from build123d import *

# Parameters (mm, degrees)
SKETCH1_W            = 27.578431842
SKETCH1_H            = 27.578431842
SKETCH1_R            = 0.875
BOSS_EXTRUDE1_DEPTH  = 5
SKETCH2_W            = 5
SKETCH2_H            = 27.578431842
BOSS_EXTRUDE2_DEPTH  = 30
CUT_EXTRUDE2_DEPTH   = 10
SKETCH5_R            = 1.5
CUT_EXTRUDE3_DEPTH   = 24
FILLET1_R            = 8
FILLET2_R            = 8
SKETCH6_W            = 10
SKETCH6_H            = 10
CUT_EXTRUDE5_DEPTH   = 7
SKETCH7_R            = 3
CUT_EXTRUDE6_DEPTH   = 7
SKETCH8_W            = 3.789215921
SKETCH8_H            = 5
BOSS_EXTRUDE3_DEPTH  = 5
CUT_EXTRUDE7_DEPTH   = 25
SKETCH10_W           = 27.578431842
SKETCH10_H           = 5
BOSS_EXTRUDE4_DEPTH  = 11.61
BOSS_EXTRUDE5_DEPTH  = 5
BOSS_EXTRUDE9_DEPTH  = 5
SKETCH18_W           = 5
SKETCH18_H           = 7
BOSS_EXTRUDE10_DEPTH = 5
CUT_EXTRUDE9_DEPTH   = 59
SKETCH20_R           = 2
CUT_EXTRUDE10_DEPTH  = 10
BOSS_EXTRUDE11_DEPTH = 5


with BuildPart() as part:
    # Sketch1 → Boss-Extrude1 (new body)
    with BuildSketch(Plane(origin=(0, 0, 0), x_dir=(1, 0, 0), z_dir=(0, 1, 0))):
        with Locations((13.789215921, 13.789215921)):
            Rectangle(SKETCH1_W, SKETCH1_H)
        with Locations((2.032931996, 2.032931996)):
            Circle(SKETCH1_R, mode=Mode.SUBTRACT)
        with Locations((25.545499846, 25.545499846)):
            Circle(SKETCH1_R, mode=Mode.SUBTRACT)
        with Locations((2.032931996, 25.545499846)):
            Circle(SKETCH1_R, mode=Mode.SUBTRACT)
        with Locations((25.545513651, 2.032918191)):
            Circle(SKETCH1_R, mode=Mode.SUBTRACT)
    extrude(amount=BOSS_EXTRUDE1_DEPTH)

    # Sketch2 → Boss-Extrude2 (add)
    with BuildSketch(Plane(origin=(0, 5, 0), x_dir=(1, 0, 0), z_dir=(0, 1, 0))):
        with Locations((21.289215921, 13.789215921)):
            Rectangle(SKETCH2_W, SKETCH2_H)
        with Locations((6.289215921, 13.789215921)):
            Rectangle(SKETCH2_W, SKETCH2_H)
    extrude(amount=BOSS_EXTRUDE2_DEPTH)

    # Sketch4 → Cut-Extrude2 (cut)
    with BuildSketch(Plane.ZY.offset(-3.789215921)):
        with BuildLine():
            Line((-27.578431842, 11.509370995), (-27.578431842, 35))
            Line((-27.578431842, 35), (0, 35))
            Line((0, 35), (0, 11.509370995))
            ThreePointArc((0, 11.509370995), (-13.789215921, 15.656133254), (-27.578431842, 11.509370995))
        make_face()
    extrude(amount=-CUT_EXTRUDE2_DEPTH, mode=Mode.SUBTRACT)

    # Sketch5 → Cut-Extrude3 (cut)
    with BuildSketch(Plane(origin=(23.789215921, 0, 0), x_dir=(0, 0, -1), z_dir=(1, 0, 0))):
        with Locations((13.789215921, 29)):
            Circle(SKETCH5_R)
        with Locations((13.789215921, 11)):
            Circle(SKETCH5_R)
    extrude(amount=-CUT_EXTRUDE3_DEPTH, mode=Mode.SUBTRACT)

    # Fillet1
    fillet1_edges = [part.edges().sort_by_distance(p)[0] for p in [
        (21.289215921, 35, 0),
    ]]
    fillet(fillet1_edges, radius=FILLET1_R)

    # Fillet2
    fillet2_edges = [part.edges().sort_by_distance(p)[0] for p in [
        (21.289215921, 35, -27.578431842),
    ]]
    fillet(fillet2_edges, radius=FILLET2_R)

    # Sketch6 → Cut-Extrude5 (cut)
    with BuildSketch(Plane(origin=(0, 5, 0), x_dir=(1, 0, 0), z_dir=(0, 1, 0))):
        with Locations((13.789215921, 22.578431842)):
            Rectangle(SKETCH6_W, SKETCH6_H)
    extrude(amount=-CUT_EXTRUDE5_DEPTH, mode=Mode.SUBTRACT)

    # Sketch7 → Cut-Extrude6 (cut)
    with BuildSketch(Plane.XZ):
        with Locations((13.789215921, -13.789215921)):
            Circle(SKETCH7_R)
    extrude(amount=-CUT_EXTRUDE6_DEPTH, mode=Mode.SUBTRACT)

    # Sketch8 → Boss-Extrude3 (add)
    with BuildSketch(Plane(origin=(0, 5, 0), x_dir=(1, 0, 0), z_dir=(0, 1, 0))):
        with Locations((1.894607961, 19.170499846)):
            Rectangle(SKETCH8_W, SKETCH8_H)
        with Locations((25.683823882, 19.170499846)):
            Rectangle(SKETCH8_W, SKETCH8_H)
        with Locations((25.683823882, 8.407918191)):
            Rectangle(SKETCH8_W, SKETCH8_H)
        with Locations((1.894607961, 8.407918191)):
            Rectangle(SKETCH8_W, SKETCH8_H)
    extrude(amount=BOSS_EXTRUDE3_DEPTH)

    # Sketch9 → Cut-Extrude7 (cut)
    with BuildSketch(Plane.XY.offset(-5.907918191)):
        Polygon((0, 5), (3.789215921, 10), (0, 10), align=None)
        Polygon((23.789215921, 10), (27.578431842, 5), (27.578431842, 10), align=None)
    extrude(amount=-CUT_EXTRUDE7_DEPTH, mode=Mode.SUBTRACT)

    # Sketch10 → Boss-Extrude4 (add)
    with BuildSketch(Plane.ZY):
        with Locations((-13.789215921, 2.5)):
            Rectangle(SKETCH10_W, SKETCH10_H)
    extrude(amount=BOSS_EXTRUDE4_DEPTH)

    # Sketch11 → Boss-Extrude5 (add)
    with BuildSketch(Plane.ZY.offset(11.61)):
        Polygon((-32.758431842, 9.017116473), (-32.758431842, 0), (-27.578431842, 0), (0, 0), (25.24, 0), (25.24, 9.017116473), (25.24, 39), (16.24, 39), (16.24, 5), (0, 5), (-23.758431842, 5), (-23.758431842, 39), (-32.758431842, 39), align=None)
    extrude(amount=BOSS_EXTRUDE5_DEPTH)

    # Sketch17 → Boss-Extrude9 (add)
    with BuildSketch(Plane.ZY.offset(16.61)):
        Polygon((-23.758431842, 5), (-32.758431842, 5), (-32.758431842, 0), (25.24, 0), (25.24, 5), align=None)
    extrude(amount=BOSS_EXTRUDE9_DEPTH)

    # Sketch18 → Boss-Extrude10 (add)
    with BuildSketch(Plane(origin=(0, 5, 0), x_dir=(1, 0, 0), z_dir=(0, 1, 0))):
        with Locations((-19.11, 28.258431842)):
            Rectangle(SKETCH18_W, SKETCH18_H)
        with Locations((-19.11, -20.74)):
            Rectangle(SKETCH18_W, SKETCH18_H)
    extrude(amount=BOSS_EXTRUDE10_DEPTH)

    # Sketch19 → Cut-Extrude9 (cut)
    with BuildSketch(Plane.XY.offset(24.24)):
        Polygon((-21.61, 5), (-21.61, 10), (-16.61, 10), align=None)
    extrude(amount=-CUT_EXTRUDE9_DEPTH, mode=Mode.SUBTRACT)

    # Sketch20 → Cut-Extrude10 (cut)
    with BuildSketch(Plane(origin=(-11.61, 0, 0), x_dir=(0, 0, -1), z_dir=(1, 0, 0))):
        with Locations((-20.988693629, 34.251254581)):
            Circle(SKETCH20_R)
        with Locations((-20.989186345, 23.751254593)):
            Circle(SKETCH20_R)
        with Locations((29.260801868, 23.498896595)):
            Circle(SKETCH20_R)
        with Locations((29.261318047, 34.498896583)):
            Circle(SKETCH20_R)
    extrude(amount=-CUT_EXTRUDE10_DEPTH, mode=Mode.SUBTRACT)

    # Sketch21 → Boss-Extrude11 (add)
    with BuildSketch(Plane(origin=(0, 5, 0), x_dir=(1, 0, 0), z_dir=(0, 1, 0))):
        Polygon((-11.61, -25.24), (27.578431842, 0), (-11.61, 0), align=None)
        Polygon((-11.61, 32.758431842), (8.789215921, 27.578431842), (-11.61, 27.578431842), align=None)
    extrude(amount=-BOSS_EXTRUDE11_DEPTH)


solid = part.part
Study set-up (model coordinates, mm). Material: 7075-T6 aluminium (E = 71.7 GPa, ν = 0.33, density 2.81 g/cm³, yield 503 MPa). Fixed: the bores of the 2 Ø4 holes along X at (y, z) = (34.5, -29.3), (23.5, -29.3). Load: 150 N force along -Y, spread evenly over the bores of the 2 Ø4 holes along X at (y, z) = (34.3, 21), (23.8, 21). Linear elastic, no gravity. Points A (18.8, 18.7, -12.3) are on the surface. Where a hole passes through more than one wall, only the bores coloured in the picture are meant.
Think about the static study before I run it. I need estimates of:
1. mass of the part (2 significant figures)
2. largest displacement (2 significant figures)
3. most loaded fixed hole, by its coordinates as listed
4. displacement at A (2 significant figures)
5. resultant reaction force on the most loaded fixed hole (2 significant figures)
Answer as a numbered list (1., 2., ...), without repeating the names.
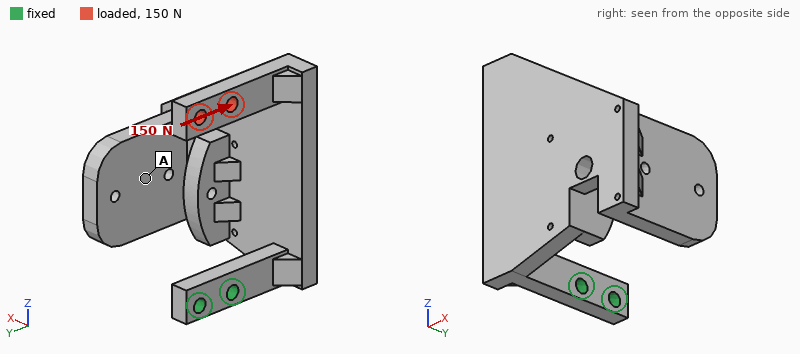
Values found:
1. 53 g
2. 0.81 mm
3. (34.5, -29.3)
4. 0.19 mm
5. 310 N
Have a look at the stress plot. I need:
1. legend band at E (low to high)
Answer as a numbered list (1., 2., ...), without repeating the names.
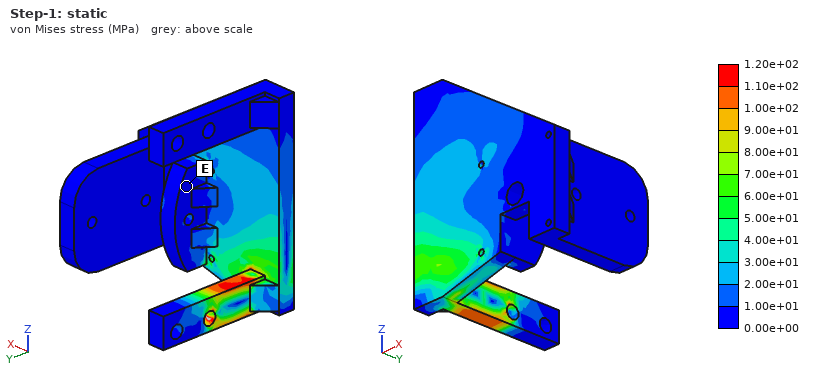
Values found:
1. 0.00e+00 to 1.00e+01 MPa
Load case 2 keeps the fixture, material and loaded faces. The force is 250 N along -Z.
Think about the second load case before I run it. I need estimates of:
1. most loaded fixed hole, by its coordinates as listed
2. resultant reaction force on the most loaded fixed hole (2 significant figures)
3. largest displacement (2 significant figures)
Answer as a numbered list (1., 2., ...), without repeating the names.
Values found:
1. (23.5, -29.3)
2. 210 N
3. 0.94 mm
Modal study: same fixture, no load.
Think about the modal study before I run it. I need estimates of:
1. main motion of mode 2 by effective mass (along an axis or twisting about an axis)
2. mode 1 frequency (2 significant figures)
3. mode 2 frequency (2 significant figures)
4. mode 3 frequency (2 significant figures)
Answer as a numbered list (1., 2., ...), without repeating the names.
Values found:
1. along Y
2. 410 Hz
3. 480 Hz
4. 750 Hz
